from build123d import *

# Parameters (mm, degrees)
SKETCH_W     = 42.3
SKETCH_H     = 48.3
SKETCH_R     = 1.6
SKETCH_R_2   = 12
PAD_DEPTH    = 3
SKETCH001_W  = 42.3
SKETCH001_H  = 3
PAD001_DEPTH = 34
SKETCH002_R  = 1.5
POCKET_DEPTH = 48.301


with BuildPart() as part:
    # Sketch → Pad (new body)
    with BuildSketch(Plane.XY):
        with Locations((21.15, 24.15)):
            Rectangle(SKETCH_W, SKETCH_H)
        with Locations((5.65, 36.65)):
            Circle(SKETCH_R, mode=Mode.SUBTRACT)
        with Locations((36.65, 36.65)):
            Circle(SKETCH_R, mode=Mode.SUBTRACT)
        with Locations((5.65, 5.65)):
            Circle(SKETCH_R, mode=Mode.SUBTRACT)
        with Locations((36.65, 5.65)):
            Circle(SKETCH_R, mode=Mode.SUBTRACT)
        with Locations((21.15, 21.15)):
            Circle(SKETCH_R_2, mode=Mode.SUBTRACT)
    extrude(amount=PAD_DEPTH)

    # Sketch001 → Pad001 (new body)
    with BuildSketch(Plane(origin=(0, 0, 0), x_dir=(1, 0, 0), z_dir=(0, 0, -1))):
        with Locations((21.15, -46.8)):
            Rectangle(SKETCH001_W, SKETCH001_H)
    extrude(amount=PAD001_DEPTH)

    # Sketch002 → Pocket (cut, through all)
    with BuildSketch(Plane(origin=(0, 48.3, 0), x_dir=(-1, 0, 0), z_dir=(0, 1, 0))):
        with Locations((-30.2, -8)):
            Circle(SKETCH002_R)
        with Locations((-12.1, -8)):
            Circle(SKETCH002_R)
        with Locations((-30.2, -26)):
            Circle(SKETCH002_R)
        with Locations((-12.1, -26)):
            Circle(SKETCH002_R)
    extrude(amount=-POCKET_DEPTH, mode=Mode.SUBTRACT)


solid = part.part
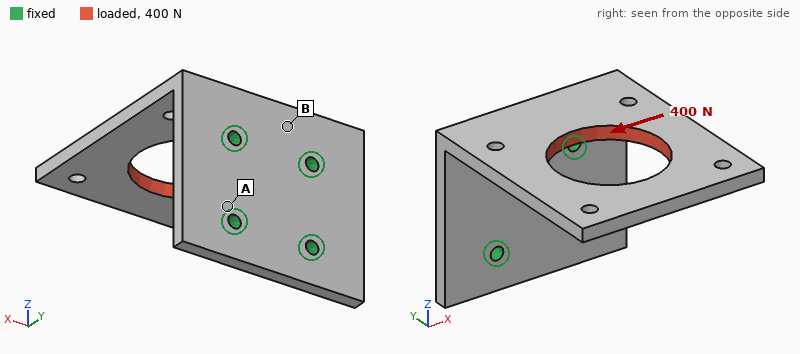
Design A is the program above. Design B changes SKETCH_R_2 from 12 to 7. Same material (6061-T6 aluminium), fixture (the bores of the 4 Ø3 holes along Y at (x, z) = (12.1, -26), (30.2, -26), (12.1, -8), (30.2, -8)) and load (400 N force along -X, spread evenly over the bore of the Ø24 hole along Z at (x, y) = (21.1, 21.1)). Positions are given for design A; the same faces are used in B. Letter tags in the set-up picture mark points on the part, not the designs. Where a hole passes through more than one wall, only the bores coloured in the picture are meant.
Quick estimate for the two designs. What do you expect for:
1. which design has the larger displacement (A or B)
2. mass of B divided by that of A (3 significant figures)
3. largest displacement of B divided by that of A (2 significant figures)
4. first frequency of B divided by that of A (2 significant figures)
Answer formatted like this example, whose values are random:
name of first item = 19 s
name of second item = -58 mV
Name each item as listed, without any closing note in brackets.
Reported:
which design has the larger displacement = A
mass of B divided by that of A = 1.10
largest displacement of B divided by that of A = 0.92
first frequency of B divided by that of A = 1.00
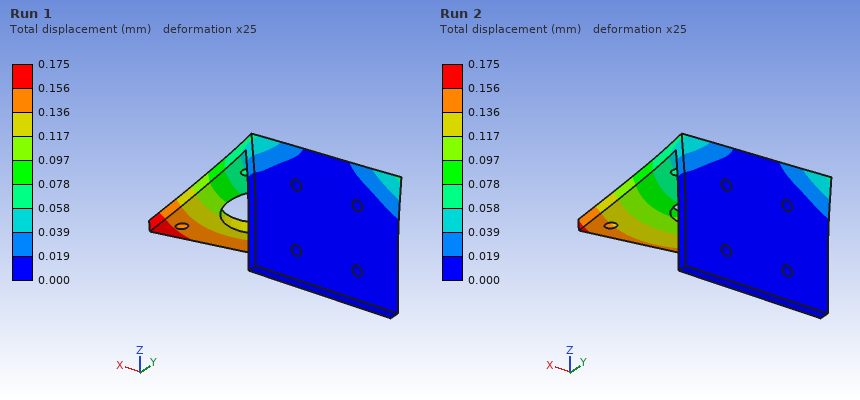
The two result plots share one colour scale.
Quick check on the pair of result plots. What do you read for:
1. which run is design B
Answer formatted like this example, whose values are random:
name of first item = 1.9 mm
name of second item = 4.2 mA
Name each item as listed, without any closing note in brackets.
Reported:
which run is design B = Run 2
